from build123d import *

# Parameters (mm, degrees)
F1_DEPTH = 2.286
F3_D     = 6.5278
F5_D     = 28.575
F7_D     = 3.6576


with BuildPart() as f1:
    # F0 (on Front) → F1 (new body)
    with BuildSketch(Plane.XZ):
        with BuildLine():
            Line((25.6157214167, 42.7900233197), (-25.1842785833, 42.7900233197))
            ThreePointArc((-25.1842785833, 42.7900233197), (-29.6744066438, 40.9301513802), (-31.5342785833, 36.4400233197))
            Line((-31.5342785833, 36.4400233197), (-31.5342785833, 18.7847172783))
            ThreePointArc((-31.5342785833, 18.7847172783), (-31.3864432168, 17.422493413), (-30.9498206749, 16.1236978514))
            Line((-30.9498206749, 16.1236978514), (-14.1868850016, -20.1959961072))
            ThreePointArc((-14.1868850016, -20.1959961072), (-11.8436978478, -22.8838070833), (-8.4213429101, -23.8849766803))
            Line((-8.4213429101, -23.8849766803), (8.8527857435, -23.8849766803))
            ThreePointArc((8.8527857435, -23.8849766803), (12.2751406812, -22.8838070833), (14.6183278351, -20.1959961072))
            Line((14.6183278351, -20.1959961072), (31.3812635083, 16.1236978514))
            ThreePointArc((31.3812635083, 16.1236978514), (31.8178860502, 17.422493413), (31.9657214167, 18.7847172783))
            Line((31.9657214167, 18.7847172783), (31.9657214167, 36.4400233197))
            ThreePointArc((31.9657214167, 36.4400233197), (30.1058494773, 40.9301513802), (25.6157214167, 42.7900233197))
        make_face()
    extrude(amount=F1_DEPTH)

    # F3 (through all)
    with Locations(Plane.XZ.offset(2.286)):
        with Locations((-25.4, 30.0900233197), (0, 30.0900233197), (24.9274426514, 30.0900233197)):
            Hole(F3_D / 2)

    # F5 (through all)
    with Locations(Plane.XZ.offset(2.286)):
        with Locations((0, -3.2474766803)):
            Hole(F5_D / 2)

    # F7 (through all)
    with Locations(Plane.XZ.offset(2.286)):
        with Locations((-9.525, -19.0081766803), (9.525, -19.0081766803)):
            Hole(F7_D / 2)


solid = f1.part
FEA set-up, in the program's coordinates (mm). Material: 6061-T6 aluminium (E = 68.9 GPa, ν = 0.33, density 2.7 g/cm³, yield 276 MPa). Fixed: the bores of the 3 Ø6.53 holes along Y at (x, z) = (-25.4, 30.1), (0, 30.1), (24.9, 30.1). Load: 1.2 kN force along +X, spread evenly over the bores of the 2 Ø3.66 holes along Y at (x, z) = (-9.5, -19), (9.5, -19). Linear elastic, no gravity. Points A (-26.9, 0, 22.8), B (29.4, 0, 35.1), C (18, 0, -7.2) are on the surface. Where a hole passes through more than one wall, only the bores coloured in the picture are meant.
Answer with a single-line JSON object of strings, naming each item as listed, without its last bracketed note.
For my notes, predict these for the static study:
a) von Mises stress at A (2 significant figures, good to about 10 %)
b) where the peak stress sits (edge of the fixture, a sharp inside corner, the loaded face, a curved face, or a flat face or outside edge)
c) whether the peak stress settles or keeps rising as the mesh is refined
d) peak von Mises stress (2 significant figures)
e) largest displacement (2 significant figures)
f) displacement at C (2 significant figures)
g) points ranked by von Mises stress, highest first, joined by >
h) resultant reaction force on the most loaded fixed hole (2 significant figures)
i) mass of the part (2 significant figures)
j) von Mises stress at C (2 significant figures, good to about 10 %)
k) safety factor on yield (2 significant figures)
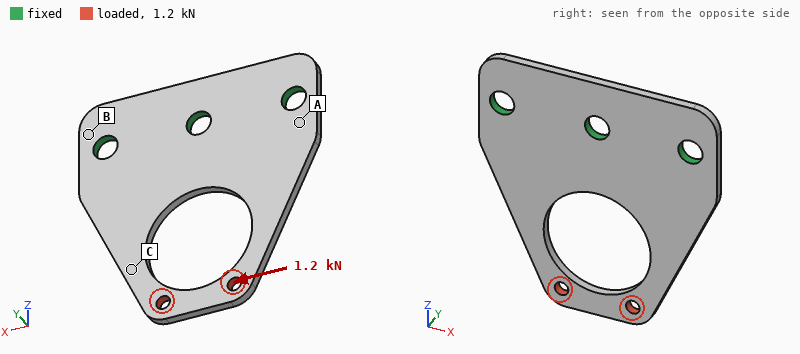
{"von Mises stress at A": "44 MPa", "where the peak stress sits": "a curved face", "whether the peak stress settles or keeps rising as the mesh is refined": "settles", "peak von Mises stress": "260 MPa", "largest displacement": "0.14 mm", "displacement at C": "0.077 mm", "points ranked by von Mises stress, highest first, joined by >": "C > A > B", "resultant reaction force on the most loaded fixed hole": "1.1 kN", "mass of the part": "16 g", "von Mises stress at C": "83 MPa", "safety factor on yield": "1.1"}
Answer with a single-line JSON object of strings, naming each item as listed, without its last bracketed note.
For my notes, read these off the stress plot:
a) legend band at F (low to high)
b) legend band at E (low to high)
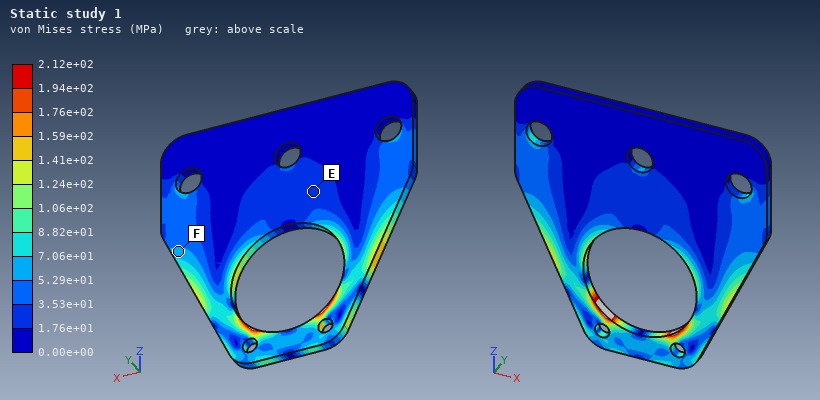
{"legend band at F": "5.29e+01 to 7.06e+01 MPa", "legend band at E": "1.76e+01 to 3.53e+01 MPa"}
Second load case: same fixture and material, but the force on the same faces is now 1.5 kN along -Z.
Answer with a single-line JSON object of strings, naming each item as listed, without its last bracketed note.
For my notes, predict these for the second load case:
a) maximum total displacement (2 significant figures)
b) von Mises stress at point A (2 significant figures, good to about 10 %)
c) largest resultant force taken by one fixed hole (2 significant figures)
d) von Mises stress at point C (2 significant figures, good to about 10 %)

{"maximum total displacement": "52 µm", "von Mises stress at point A": "28 MPa", "largest resultant force taken by one fixed hole": "730 N", "von Mises stress at point C": "38 MPa"}
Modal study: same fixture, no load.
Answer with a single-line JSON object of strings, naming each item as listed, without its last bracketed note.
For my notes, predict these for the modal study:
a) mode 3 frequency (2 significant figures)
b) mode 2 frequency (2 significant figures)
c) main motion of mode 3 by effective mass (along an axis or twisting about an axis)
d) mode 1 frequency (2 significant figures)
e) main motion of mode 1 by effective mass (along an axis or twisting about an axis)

{"mode 3 frequency": "4000 Hz", "mode 2 frequency": "2400 Hz", "main motion of mode 3 by effective mass": "along Y", "mode 1 frequency": "1000 Hz", "main motion of mode 1 by effective mass": "along Y"}
